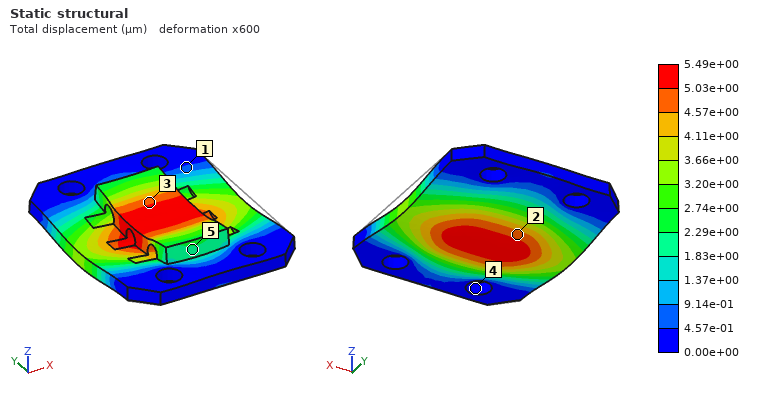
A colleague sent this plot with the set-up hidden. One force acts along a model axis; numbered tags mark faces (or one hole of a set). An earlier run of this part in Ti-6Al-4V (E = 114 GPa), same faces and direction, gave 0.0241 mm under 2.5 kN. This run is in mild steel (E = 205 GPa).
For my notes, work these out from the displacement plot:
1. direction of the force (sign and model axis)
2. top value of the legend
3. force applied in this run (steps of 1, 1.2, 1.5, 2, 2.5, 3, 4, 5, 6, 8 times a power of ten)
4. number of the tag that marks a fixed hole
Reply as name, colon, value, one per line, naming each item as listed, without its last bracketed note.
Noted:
direction of the force: -Z
top value of the legend: 5.49e+00 µm
force applied in this run: 1 kN
number of the tag that marks a fixed hole: 4
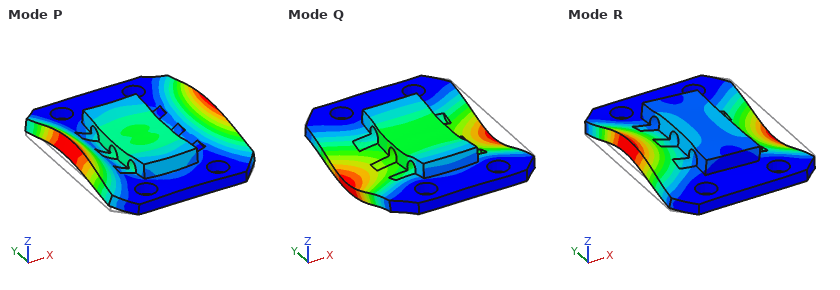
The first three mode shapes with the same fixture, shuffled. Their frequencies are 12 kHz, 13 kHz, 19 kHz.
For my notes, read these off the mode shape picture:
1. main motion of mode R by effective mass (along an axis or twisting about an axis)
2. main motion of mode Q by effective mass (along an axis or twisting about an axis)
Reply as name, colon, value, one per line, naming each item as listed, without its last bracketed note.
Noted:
main motion of mode R by effective mass: twisting about Y
main motion of mode Q by effective mass: along Z
